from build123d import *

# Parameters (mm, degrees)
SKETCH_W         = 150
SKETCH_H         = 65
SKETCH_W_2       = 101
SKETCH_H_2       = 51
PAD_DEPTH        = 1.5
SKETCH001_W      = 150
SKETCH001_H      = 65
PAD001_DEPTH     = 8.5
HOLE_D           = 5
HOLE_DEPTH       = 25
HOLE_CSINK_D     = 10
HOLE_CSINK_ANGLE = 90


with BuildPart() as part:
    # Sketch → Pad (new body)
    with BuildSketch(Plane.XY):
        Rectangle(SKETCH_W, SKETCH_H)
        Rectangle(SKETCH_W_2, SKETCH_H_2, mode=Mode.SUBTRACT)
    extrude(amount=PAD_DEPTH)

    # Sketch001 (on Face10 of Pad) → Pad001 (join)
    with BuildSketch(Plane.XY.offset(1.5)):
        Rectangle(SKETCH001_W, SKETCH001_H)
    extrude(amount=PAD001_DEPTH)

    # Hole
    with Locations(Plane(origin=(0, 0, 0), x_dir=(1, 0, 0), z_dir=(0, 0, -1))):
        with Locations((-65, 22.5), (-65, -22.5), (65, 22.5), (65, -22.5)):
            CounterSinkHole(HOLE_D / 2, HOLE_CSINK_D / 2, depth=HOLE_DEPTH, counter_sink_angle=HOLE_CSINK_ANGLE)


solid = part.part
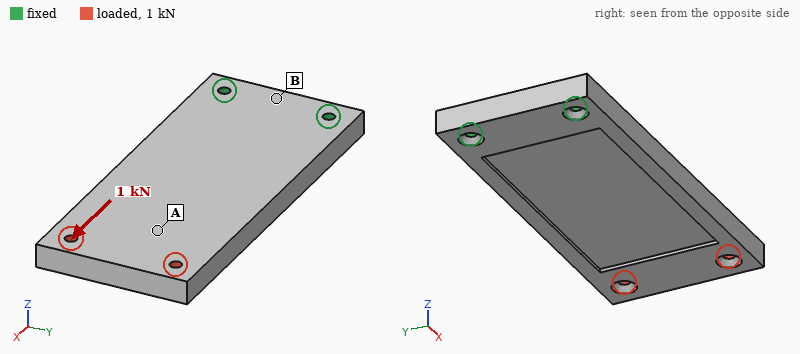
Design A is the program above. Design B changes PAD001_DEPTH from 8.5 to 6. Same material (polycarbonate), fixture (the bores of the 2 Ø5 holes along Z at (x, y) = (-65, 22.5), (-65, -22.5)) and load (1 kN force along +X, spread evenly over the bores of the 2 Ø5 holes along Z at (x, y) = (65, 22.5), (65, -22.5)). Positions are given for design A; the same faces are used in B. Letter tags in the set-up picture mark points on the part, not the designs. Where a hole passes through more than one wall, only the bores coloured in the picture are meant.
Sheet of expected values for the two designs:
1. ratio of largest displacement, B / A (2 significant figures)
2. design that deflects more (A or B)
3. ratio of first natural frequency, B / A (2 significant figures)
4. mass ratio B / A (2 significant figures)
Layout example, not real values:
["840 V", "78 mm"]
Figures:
["2.5", "B", "0.74", "0.73"]
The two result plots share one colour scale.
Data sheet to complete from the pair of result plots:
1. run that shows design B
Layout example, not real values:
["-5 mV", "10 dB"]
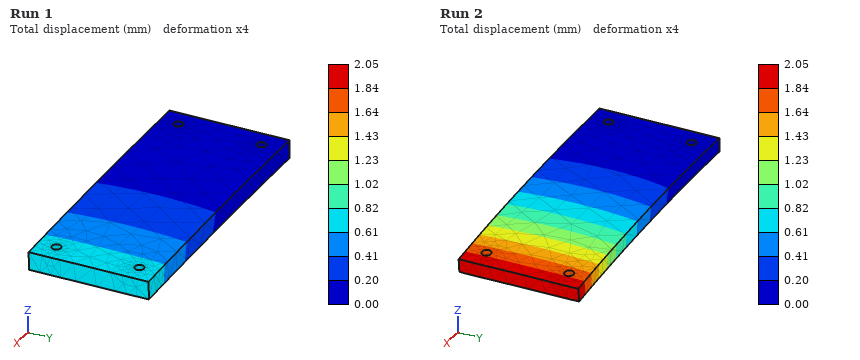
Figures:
["Run 2"]
